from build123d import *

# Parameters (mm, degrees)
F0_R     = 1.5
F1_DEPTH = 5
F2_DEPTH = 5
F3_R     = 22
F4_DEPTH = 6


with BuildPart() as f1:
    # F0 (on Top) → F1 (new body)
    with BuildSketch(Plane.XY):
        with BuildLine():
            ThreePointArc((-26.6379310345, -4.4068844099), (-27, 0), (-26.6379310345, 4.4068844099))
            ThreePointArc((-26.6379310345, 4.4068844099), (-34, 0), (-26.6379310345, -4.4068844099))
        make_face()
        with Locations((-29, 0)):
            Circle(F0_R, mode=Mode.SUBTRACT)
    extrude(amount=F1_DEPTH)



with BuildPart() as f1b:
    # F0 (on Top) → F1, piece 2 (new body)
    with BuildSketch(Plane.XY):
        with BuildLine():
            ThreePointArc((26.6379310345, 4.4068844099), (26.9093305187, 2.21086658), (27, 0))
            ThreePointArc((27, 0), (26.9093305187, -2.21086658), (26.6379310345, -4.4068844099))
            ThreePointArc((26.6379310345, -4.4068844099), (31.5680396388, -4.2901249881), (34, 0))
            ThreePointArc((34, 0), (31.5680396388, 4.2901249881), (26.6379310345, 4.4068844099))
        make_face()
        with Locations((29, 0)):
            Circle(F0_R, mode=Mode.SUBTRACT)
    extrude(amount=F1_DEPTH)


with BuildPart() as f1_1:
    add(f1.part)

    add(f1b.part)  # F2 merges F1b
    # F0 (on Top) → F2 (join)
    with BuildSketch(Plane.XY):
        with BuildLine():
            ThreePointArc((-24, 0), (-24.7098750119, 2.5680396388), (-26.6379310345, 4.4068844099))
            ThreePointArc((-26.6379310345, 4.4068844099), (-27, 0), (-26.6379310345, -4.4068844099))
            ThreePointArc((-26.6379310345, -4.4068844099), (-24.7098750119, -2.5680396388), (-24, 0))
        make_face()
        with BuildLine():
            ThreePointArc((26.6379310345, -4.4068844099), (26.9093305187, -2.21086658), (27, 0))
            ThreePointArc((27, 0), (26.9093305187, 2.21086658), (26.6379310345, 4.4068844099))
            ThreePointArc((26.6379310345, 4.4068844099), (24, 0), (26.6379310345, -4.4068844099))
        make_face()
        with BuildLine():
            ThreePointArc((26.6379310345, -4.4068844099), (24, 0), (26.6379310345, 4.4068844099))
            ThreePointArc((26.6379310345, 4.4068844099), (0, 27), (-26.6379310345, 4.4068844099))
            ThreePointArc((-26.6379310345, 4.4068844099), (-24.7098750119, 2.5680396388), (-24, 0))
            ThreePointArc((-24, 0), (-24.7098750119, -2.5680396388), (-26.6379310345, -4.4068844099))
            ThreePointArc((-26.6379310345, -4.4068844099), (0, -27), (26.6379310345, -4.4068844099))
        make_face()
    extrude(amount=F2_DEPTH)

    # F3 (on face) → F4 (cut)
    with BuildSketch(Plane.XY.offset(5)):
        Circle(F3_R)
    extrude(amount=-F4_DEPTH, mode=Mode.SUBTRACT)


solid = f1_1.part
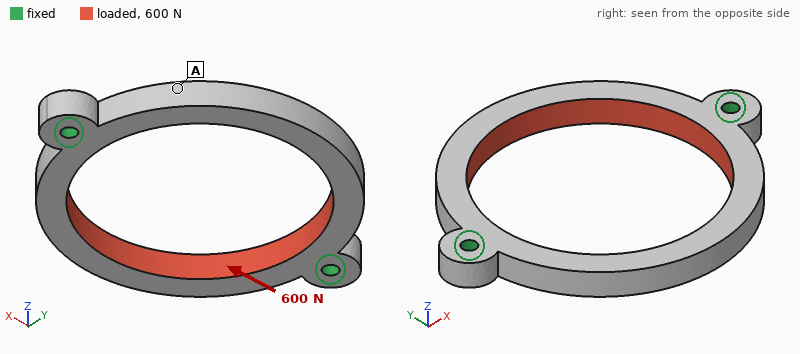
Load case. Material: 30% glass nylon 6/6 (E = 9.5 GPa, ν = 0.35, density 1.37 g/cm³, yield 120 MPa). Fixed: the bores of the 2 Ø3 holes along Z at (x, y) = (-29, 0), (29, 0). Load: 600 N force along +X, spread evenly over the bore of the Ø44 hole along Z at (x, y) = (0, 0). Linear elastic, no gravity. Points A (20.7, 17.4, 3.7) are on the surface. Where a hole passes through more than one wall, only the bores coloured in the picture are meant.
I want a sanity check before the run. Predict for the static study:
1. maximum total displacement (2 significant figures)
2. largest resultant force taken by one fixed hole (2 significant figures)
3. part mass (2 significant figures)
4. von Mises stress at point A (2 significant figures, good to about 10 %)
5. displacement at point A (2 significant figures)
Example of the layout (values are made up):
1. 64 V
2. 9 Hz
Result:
1. 0.14 mm
2. 300 N
3. 6.0 g
4. 12 MPa
5. 0.12 mm
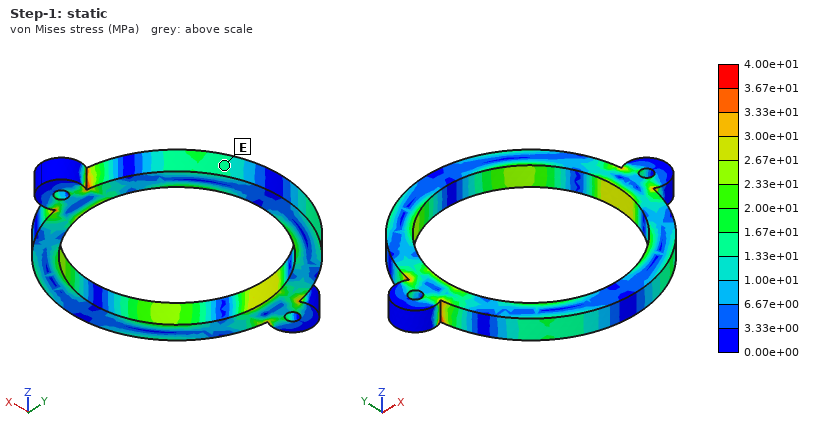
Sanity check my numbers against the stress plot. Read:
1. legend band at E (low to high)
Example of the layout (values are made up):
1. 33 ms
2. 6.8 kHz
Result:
1. 1.33e+01 to 1.67e+01 MPa
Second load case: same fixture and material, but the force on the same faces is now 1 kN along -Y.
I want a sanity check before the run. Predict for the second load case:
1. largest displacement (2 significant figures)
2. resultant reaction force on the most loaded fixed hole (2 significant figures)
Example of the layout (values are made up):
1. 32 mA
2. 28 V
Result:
1. 59 µm
2. 500 N
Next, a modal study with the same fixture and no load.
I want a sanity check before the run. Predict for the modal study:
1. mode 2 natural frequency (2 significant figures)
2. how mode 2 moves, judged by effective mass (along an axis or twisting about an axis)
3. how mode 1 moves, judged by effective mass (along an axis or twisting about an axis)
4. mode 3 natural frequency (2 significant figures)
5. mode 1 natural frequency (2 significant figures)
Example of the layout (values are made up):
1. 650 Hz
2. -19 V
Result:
1. 1900 Hz
2. along Z
3. twisting about X
4. 4100 Hz
5. 1700 Hz
